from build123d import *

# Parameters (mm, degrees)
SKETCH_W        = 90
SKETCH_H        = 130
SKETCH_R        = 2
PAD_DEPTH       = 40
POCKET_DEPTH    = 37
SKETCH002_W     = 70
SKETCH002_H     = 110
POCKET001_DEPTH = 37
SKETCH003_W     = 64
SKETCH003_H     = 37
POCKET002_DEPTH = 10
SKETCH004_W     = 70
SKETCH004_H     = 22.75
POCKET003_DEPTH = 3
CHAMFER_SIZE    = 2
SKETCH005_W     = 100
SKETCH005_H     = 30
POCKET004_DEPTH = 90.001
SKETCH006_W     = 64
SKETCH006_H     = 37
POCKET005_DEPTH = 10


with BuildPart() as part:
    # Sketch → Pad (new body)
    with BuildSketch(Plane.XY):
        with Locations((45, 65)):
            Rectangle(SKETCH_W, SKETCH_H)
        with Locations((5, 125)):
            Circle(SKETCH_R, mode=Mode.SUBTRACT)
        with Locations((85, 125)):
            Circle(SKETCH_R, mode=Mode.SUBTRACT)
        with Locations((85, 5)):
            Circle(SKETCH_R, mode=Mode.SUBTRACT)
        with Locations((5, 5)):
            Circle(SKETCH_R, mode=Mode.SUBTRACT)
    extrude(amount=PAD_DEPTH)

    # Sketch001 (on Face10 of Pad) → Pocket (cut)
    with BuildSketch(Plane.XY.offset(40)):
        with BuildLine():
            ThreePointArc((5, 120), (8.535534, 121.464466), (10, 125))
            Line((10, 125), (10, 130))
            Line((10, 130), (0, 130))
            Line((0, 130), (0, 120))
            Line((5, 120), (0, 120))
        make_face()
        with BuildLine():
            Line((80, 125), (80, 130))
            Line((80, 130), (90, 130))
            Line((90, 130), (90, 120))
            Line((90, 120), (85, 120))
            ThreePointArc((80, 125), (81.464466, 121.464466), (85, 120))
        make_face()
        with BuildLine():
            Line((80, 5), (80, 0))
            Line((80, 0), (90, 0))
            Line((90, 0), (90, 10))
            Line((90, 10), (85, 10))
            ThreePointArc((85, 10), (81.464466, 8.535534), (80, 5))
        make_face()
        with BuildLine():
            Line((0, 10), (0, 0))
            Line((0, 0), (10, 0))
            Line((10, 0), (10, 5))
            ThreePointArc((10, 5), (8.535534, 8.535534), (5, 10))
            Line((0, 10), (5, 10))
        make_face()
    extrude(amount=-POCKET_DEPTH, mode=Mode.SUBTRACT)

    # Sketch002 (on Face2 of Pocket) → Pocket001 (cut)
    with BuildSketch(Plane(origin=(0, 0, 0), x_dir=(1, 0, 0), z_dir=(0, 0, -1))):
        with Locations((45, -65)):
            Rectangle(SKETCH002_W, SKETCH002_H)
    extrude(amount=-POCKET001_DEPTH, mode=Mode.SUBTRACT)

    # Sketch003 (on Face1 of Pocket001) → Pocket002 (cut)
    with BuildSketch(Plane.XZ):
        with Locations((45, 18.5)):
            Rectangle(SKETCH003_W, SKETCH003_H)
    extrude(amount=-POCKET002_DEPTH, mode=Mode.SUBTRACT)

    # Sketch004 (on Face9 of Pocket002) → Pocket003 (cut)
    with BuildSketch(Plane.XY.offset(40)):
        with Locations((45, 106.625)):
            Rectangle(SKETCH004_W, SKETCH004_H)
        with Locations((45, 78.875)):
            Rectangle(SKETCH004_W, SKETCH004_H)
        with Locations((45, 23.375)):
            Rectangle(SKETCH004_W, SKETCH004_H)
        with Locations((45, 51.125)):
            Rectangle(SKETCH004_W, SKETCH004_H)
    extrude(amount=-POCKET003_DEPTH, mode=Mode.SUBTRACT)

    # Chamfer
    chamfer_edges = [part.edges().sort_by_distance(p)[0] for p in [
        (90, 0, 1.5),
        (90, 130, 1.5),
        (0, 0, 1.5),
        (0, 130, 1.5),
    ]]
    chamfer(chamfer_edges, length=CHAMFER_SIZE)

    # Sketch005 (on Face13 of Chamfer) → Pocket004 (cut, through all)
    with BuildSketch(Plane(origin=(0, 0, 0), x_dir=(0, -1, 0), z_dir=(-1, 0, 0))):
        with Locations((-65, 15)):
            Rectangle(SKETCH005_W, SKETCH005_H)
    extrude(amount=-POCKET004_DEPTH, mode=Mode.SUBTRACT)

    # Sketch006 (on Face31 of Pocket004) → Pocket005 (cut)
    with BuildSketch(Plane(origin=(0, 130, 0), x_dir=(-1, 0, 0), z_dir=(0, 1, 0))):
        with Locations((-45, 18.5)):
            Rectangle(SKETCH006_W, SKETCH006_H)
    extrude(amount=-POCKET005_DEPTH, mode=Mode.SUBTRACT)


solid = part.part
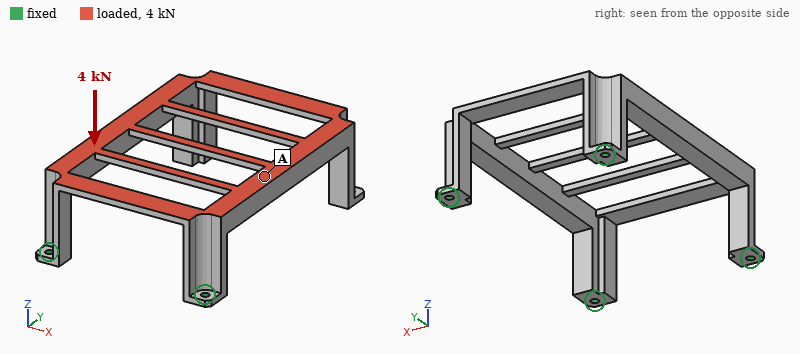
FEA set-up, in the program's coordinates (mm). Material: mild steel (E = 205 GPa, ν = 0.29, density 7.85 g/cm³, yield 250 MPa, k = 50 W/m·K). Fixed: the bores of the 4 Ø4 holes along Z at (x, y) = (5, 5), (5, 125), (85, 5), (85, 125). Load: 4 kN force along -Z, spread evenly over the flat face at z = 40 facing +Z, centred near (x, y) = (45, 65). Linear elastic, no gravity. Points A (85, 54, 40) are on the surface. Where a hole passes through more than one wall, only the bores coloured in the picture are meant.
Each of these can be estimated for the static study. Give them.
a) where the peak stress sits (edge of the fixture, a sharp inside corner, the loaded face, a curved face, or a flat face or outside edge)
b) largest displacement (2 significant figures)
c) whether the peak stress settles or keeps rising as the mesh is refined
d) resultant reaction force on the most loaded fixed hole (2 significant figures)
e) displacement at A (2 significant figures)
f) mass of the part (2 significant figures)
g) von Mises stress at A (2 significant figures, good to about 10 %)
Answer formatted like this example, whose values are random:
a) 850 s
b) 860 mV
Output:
a) edge of the fixture
b) 0.22 mm
c) keeps rising
d) 1.1 kN
e) 0.053 mm
f) 330 g
g) 53 MPa
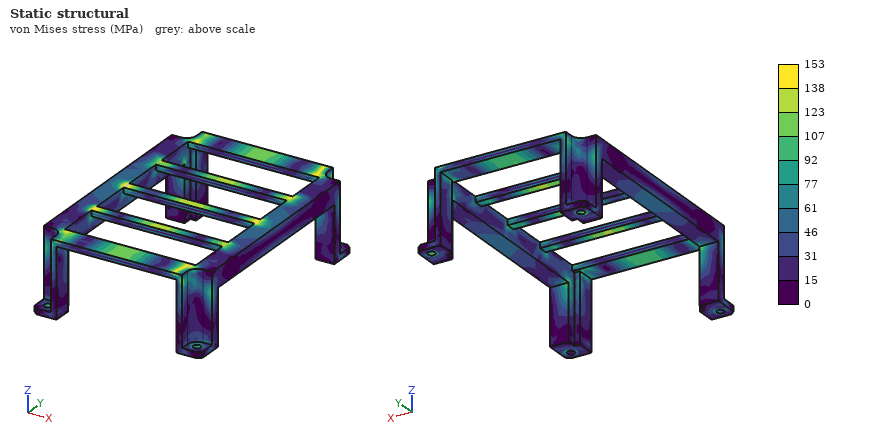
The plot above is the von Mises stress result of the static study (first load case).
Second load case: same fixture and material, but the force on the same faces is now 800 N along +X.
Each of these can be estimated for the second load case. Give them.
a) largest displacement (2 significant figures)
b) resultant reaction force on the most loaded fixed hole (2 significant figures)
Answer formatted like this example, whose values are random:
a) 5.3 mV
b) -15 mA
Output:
a) 90 µm
b) 210 N
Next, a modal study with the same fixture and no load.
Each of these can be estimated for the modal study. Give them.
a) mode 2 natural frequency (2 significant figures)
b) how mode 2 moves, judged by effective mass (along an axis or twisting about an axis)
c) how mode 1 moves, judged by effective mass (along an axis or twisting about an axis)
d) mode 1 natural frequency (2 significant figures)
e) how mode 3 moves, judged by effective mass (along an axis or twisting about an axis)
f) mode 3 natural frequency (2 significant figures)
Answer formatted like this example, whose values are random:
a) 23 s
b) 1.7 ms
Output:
a) 1700 Hz
b) along Y
c) along X
d) 1000 Hz
e) twisting about Z
f) 1900 Hz
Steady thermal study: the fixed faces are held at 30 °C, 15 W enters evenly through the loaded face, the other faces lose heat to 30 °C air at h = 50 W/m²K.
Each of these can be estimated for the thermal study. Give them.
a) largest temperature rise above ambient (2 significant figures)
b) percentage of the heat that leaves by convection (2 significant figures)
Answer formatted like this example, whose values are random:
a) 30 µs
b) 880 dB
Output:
a) 20 K
b) 73 %
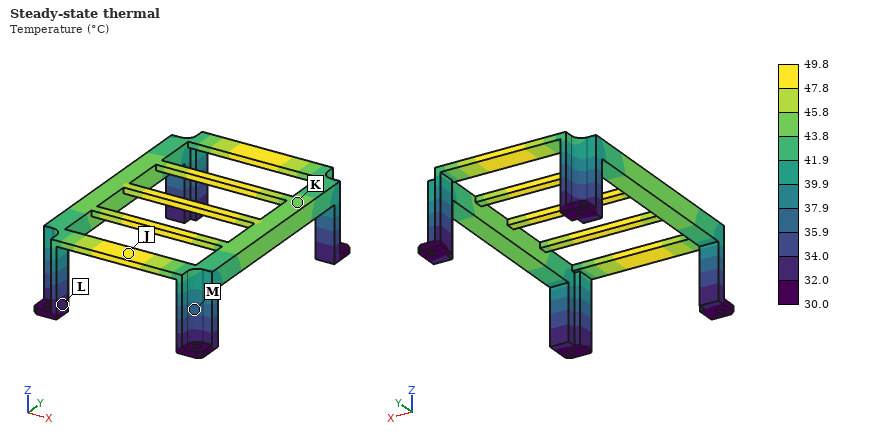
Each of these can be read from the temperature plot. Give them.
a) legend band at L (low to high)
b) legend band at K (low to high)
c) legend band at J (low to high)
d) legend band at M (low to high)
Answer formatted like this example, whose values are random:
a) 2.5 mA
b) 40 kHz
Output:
a) 32.0 to 34.0 °C
b) 43.8 to 45.8 °C
c) 47.8 to 49.8 °C
d) 35.9 to 37.9 °C
